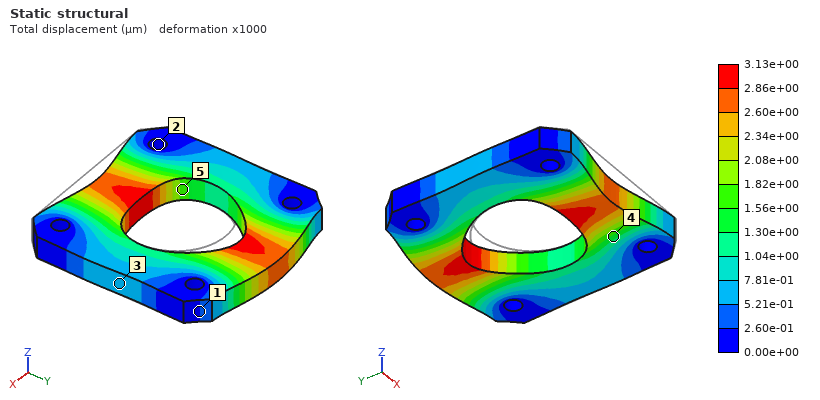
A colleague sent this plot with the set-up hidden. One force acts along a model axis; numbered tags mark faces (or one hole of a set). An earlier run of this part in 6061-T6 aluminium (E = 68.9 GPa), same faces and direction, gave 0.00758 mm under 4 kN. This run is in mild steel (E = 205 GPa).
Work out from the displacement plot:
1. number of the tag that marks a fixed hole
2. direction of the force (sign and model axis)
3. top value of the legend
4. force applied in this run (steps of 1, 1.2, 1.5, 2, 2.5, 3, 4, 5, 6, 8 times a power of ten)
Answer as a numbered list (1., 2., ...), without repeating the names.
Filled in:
1. 2
2. +Y
3. 3.13e+00 µm
4. 5 kN
